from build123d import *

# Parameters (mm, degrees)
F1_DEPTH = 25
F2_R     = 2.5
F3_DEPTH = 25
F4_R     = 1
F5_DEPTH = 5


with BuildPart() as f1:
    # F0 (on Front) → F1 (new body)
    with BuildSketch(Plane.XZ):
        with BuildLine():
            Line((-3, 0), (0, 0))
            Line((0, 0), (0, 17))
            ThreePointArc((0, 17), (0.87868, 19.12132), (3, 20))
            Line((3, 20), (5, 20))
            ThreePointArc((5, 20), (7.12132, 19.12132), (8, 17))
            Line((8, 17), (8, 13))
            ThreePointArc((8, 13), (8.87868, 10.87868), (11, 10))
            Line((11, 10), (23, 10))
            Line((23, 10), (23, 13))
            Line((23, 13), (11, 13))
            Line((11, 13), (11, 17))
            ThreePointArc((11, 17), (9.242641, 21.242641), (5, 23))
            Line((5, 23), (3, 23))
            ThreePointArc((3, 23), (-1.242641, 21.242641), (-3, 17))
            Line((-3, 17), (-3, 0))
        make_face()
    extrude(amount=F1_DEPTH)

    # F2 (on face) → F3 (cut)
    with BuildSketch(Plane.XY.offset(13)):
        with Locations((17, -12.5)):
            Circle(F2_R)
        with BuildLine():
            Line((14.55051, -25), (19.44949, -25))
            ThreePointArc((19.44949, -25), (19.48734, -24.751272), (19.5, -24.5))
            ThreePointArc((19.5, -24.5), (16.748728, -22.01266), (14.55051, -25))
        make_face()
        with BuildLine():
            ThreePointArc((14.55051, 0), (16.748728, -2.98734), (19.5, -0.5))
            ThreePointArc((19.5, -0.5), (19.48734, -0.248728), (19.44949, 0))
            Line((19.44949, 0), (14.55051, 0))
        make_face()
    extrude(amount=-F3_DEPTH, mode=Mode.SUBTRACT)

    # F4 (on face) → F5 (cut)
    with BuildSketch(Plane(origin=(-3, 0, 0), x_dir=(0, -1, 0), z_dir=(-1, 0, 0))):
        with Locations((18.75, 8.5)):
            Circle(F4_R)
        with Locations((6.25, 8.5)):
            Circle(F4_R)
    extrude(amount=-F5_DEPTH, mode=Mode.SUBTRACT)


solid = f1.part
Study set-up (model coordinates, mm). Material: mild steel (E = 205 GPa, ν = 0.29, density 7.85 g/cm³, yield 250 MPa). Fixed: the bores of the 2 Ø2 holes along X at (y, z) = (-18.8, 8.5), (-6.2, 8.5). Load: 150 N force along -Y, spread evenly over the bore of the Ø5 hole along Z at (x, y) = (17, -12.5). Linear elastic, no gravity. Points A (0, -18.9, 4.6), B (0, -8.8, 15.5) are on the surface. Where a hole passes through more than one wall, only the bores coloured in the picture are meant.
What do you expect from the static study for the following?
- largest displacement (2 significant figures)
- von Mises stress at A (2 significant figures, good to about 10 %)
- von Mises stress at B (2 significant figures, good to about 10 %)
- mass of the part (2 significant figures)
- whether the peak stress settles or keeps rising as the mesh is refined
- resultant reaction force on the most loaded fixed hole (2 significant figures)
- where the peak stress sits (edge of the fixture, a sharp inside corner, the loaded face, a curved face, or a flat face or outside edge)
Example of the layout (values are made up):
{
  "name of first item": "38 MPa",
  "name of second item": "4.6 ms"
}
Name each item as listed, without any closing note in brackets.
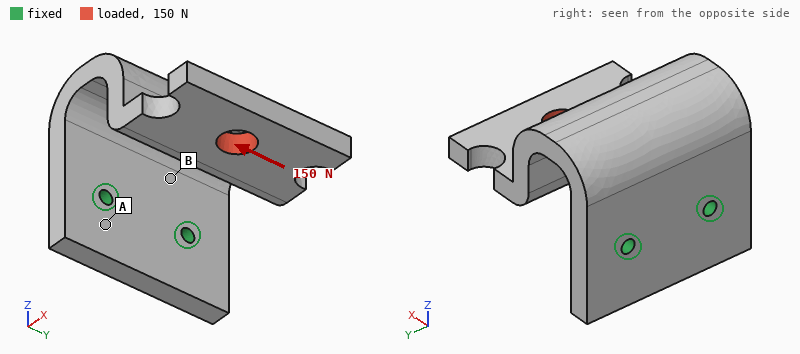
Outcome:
{
  "largest displacement": "43 µm",
  "von Mises stress at A": "8.7 MPa",
  "von Mises stress at B": "49 MPa",
  "mass of the part": "29 g",
  "whether the peak stress settles or keeps rising as the mesh is refined": "keeps rising",
  "resultant reaction force on the most loaded fixed hole": "190 N",
  "where the peak stress sits": "edge of the fixture"
}
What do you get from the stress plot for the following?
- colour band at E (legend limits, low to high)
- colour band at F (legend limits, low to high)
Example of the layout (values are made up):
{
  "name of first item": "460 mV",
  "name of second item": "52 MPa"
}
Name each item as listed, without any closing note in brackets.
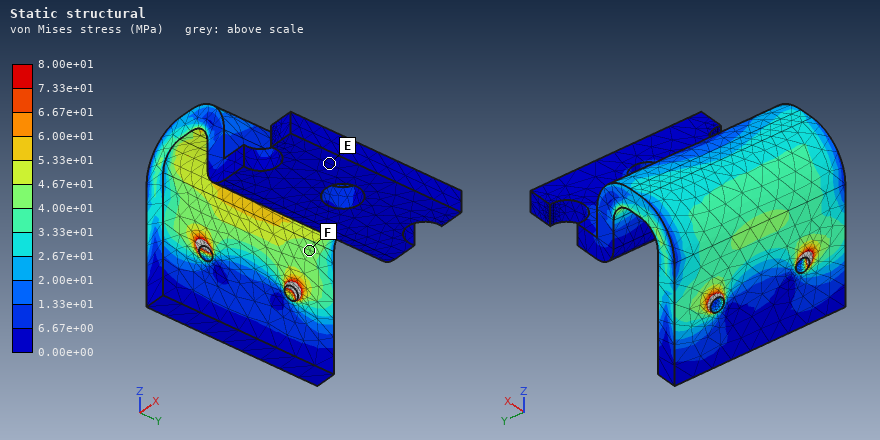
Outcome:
{
  "colour band at E": "0.00e+00 to 6.67e+00 MPa",
  "colour band at F": "4.00e+01 to 4.67e+01 MPa"
}
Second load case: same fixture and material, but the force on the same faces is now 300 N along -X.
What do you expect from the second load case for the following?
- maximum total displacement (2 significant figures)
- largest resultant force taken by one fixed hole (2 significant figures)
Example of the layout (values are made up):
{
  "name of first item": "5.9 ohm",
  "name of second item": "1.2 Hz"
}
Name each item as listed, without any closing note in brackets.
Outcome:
{
  "maximum total displacement": "85 µm",
  "largest resultant force taken by one fixed hole": "150 N"
}
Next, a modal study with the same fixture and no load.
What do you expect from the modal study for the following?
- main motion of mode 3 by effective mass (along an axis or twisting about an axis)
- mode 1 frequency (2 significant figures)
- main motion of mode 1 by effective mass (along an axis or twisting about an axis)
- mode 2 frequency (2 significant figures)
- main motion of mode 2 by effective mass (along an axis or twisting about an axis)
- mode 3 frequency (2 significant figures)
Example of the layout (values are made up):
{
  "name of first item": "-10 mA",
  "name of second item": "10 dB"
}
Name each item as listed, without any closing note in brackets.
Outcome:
{
  "main motion of mode 3 by effective mass": "along X",
  "mode 1 frequency": "2200 Hz",
  "main motion of mode 1 by effective mass": "along Z",
  "mode 2 frequency": "3500 Hz",
  "main motion of mode 2 by effective mass": "along Y",
  "mode 3 frequency": "5300 Hz"
}
